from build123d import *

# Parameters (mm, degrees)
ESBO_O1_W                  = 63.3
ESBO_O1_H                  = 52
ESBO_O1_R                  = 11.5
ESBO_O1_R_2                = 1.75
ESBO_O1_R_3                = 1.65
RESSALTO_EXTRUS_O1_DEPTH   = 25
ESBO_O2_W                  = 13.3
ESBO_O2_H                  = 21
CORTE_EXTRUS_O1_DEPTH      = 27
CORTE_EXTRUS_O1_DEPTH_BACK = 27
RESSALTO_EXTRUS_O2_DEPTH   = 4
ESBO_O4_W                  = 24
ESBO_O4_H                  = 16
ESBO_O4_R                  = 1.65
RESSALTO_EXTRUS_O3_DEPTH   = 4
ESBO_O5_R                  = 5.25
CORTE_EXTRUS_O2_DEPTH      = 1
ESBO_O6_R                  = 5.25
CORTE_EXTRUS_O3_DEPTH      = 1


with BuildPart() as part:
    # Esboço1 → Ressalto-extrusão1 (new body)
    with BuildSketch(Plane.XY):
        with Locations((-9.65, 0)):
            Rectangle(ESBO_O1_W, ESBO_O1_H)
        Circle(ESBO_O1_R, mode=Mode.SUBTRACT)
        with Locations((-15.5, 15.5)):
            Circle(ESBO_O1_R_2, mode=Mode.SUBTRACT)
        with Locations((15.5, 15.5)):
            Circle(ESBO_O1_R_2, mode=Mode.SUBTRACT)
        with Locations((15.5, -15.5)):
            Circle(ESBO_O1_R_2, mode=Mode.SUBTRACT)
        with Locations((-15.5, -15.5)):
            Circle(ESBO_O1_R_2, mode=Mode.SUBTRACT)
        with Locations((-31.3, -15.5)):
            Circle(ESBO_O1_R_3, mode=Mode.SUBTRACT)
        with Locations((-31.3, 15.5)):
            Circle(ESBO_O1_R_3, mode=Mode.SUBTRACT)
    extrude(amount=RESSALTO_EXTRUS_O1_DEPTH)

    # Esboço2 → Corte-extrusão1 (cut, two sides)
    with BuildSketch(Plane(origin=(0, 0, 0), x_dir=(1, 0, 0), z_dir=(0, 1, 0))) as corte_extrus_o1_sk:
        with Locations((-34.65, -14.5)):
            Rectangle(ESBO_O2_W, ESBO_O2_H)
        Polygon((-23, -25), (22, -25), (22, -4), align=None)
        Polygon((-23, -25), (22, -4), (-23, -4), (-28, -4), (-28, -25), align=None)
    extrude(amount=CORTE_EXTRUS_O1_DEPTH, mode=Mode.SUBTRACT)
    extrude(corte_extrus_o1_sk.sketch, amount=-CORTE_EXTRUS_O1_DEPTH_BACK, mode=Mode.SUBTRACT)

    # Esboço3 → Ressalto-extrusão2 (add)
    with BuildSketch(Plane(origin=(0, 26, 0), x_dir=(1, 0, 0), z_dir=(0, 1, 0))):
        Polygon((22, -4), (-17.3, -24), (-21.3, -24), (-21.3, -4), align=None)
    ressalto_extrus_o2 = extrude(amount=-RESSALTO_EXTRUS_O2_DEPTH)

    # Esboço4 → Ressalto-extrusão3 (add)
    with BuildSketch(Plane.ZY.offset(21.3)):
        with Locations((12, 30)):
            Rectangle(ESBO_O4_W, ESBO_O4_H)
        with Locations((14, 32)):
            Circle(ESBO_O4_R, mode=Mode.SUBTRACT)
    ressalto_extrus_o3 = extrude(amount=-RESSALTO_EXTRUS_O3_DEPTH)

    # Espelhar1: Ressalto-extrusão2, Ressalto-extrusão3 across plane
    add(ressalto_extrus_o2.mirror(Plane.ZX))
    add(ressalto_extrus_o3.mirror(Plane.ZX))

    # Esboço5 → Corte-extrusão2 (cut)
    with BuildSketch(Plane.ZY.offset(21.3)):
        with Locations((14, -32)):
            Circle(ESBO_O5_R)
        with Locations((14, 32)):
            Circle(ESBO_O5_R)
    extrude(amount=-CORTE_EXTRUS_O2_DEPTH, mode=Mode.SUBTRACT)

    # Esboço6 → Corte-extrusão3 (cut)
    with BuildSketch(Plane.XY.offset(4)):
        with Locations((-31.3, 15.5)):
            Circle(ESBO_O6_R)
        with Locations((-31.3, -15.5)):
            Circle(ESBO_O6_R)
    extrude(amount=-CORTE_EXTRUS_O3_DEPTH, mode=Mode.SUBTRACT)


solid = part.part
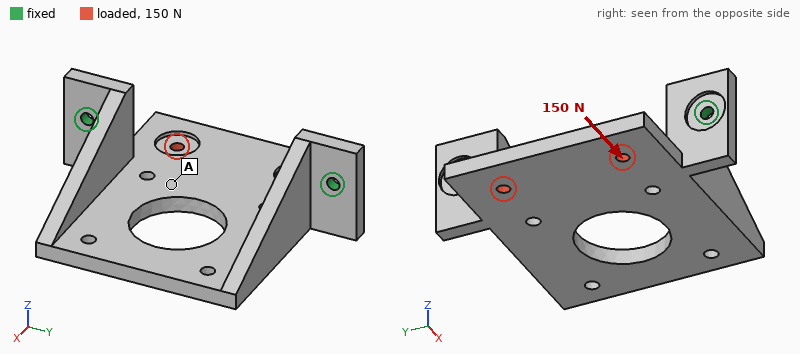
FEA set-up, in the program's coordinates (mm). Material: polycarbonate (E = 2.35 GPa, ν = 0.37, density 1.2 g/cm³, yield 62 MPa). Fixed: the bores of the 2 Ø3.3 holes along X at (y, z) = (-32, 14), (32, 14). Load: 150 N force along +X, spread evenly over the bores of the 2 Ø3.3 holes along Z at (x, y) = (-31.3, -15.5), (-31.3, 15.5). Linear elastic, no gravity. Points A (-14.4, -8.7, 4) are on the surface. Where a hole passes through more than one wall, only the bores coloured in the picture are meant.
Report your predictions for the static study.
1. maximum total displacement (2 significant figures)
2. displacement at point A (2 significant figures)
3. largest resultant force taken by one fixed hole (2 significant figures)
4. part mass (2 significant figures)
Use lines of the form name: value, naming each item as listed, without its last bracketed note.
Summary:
maximum total displacement: 1.2 mm
displacement at point A: 0.34 mm
largest resultant force taken by one fixed hole: 75 N
part mass: 20 g
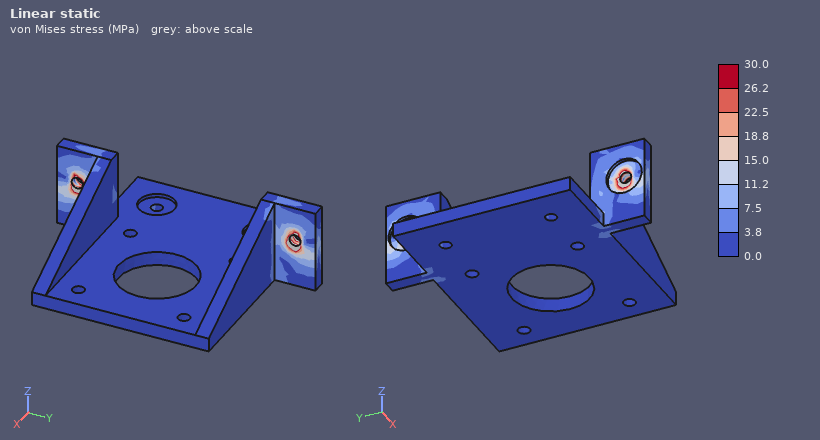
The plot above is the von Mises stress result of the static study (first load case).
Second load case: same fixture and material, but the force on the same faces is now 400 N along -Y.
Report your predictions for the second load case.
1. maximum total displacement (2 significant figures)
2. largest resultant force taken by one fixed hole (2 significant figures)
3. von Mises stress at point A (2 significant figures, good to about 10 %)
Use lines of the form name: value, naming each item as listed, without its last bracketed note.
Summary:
maximum total displacement: 0.67 mm
largest resultant force taken by one fixed hole: 220 N
von Mises stress at point A: 6.4 MPa
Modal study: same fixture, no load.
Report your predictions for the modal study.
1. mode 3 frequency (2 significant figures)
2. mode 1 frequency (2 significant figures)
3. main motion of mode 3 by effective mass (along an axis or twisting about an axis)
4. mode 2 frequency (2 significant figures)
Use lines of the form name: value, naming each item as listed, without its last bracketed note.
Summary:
mode 3 frequency: 1100 Hz
mode 1 frequency: 420 Hz
main motion of mode 3 by effective mass: along Z
mode 2 frequency: 840 Hz
